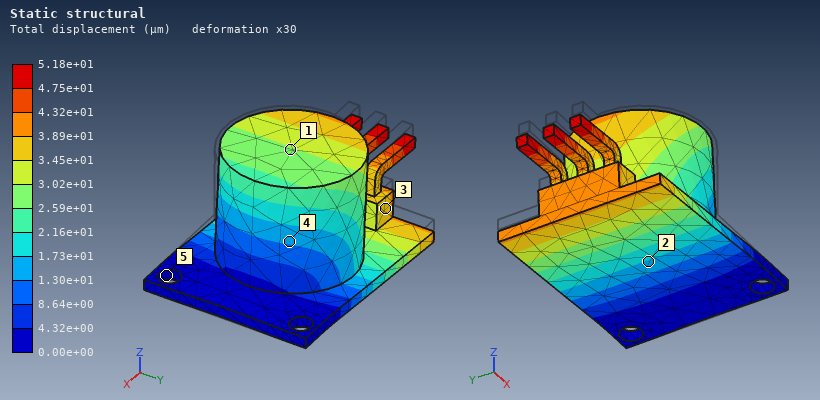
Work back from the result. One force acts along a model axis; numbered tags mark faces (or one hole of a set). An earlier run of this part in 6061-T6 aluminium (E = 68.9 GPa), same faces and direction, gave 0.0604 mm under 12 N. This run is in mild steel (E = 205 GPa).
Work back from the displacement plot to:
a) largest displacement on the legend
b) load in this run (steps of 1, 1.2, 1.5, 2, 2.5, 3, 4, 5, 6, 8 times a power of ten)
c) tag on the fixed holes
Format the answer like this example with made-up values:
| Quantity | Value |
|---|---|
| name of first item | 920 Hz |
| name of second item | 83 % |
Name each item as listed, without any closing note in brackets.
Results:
| Quantity | Value |
|---|---|
| largest displacement on the legend | 5.18e+01 µm |
| load in this run | 30 N |
| tag on the fixed holes | 5 |
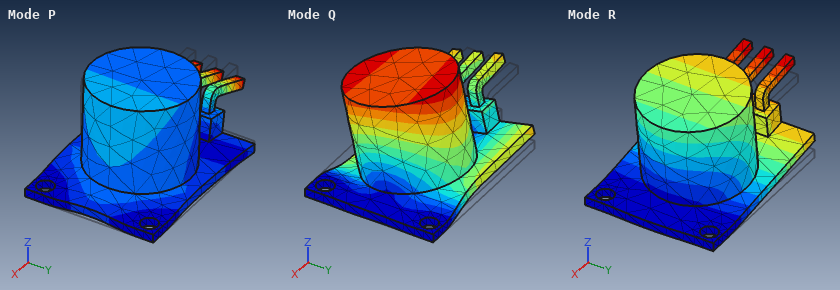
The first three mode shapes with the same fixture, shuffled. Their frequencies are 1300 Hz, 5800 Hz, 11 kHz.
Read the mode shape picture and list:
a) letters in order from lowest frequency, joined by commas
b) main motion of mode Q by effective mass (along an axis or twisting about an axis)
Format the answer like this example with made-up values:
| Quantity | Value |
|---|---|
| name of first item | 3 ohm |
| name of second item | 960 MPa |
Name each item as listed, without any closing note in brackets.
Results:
| Quantity | Value |
|---|---|
| letters in order from lowest frequency, joined by commas | R, Q, P |
| main motion of mode Q by effective mass | along Y |
